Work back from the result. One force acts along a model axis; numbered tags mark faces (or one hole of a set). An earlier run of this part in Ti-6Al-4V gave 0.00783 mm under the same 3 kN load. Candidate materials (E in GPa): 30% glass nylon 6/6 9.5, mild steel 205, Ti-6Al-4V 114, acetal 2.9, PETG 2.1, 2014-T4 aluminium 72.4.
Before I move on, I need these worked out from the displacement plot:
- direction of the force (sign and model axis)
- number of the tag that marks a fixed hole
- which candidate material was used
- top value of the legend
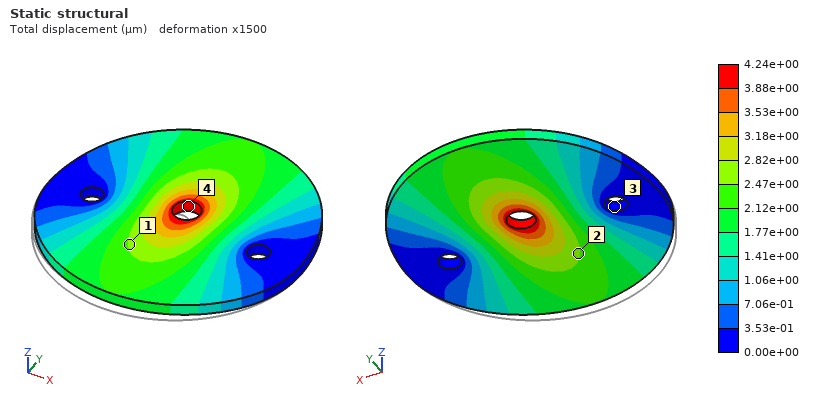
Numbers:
+Y
3
mild steel
4.24e+00 µm
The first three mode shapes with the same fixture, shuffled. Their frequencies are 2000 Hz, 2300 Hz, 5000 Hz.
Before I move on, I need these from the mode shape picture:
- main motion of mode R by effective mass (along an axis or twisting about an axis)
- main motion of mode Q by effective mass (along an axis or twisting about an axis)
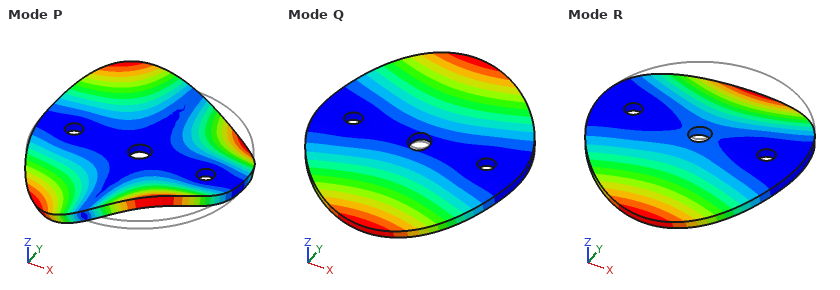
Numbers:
along Z
twisting about X
